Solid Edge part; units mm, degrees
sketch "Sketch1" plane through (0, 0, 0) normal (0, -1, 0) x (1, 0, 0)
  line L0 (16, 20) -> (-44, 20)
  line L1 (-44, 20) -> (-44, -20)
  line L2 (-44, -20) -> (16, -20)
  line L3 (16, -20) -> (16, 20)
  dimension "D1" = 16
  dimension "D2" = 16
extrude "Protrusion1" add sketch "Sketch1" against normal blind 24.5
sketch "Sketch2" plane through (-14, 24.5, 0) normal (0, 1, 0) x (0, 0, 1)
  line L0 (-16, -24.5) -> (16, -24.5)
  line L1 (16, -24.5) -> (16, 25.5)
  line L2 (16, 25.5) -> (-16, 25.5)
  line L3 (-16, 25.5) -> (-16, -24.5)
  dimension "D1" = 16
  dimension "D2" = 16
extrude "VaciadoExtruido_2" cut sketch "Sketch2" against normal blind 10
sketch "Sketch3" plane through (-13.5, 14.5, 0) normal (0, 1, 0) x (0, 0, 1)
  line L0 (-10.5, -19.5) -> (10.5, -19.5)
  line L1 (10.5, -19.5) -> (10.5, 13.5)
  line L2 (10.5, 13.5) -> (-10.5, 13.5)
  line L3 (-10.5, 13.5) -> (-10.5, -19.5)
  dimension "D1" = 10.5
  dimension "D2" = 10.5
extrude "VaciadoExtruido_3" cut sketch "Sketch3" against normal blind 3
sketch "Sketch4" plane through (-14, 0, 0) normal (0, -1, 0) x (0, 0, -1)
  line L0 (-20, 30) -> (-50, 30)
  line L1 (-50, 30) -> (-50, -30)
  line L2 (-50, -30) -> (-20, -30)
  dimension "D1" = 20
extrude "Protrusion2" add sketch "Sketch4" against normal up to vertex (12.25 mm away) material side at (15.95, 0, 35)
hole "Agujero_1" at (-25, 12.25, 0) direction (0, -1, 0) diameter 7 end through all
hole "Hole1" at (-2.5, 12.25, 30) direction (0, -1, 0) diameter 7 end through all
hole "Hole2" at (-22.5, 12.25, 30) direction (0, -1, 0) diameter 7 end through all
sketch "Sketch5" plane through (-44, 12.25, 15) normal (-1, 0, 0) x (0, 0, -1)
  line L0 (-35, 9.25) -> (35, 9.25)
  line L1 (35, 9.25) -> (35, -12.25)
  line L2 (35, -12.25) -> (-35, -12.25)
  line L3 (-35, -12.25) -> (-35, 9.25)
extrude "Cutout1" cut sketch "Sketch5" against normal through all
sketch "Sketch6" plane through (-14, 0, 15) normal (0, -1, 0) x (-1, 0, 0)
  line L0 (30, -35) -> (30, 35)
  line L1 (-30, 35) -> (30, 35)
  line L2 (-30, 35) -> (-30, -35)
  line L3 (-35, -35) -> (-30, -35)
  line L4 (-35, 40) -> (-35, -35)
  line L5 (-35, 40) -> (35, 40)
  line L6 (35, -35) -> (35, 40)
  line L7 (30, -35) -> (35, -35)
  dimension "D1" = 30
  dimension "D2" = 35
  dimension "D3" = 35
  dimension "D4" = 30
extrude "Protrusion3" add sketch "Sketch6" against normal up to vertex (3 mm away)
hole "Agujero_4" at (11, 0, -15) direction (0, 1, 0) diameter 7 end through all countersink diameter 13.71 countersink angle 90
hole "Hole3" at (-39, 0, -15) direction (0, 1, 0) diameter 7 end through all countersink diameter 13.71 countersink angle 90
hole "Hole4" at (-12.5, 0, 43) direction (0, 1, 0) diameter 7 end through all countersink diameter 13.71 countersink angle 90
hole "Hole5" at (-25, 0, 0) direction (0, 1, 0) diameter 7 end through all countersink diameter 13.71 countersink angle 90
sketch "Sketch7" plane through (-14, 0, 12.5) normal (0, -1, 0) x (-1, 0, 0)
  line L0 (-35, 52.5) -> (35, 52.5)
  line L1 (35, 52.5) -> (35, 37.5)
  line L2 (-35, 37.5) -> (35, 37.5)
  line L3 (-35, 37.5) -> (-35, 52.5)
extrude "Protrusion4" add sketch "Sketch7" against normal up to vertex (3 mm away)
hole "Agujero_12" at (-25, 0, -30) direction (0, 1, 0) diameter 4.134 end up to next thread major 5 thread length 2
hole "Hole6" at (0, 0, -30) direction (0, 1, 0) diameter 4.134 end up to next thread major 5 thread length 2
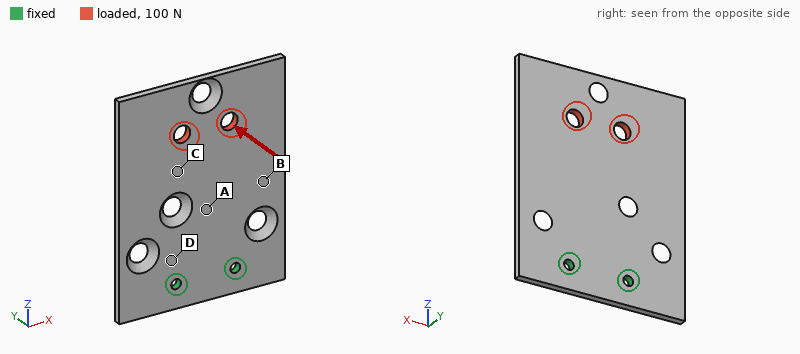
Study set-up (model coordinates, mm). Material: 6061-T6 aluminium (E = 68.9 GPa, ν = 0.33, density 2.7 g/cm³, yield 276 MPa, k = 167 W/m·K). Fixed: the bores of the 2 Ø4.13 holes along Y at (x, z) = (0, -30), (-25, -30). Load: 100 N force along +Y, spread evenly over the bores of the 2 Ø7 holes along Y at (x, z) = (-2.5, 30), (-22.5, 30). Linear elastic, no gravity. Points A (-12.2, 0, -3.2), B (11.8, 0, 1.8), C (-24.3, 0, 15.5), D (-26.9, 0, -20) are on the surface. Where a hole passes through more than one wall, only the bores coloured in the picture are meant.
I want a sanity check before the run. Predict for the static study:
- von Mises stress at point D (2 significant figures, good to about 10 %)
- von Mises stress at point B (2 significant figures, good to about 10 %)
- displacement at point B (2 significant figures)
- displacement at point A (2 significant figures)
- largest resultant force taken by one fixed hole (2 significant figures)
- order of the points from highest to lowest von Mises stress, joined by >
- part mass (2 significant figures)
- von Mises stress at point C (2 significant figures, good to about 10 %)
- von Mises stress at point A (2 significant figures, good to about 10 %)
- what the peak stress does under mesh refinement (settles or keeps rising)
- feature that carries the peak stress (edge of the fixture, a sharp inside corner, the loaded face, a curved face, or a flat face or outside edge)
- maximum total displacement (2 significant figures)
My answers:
57 MPa
25 MPa
0.29 mm
0.22 mm
52 N
D > A > B > C
47 g
12 MPa
42 MPa
keeps rising
edge of the fixture
1.3 mm
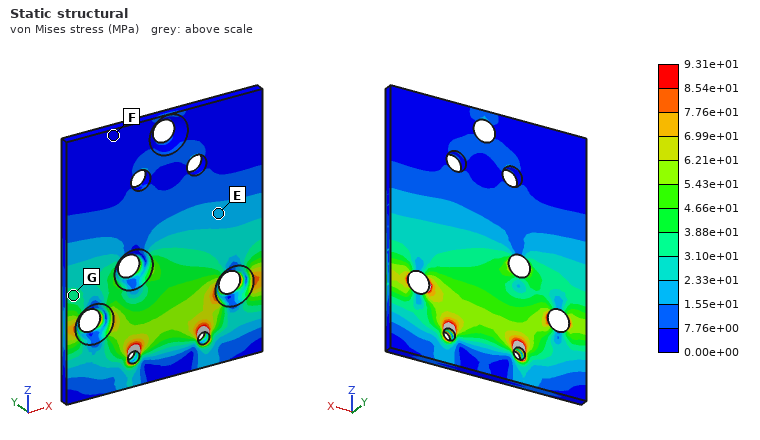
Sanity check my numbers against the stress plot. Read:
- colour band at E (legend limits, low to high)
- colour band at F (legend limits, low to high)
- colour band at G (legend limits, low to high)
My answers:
1.55e+01 to 2.33e+01 MPa
0.00e+00 to 7.76e+00 MPa
3.10e+01 to 3.88e+01 MPa
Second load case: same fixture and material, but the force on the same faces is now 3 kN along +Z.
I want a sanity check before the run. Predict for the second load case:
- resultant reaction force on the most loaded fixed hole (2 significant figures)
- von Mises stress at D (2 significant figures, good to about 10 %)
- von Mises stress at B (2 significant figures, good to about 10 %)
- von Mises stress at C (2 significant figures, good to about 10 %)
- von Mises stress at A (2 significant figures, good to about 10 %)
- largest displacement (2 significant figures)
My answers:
1.5 kN
27 MPa
9.0 MPa
16 MPa
28 MPa
44 µm
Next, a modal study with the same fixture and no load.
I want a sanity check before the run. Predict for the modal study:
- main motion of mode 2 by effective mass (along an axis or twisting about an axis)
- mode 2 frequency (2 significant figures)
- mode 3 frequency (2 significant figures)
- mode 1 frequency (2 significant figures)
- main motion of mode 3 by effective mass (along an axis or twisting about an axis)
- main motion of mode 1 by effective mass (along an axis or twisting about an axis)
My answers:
twisting about Z
890 Hz
2200 Hz
360 Hz
along Y
along Y
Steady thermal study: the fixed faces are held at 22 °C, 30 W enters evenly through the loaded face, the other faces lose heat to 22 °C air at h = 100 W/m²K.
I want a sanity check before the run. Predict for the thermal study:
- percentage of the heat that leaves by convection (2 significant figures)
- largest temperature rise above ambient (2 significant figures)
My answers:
67 %
35 K
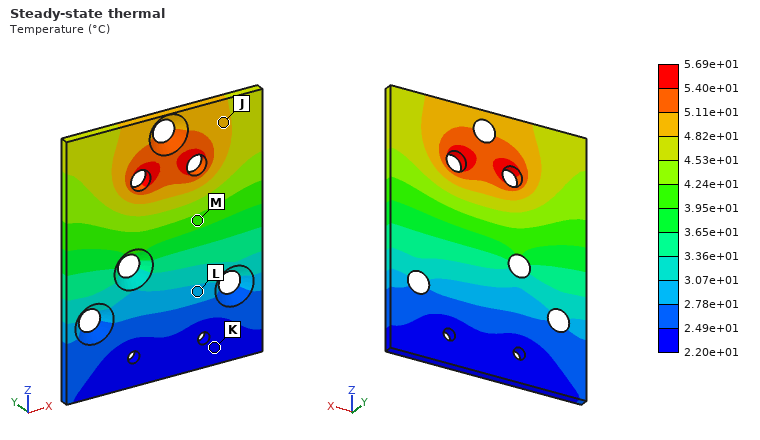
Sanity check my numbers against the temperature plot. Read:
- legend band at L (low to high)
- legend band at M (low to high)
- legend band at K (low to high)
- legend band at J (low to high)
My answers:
2.78e+01 to 3.07e+01 °C
3.95e+01 to 4.24e+01 °C
2.20e+01 to 2.49e+01 °C
4.82e+01 to 5.11e+01 °C
